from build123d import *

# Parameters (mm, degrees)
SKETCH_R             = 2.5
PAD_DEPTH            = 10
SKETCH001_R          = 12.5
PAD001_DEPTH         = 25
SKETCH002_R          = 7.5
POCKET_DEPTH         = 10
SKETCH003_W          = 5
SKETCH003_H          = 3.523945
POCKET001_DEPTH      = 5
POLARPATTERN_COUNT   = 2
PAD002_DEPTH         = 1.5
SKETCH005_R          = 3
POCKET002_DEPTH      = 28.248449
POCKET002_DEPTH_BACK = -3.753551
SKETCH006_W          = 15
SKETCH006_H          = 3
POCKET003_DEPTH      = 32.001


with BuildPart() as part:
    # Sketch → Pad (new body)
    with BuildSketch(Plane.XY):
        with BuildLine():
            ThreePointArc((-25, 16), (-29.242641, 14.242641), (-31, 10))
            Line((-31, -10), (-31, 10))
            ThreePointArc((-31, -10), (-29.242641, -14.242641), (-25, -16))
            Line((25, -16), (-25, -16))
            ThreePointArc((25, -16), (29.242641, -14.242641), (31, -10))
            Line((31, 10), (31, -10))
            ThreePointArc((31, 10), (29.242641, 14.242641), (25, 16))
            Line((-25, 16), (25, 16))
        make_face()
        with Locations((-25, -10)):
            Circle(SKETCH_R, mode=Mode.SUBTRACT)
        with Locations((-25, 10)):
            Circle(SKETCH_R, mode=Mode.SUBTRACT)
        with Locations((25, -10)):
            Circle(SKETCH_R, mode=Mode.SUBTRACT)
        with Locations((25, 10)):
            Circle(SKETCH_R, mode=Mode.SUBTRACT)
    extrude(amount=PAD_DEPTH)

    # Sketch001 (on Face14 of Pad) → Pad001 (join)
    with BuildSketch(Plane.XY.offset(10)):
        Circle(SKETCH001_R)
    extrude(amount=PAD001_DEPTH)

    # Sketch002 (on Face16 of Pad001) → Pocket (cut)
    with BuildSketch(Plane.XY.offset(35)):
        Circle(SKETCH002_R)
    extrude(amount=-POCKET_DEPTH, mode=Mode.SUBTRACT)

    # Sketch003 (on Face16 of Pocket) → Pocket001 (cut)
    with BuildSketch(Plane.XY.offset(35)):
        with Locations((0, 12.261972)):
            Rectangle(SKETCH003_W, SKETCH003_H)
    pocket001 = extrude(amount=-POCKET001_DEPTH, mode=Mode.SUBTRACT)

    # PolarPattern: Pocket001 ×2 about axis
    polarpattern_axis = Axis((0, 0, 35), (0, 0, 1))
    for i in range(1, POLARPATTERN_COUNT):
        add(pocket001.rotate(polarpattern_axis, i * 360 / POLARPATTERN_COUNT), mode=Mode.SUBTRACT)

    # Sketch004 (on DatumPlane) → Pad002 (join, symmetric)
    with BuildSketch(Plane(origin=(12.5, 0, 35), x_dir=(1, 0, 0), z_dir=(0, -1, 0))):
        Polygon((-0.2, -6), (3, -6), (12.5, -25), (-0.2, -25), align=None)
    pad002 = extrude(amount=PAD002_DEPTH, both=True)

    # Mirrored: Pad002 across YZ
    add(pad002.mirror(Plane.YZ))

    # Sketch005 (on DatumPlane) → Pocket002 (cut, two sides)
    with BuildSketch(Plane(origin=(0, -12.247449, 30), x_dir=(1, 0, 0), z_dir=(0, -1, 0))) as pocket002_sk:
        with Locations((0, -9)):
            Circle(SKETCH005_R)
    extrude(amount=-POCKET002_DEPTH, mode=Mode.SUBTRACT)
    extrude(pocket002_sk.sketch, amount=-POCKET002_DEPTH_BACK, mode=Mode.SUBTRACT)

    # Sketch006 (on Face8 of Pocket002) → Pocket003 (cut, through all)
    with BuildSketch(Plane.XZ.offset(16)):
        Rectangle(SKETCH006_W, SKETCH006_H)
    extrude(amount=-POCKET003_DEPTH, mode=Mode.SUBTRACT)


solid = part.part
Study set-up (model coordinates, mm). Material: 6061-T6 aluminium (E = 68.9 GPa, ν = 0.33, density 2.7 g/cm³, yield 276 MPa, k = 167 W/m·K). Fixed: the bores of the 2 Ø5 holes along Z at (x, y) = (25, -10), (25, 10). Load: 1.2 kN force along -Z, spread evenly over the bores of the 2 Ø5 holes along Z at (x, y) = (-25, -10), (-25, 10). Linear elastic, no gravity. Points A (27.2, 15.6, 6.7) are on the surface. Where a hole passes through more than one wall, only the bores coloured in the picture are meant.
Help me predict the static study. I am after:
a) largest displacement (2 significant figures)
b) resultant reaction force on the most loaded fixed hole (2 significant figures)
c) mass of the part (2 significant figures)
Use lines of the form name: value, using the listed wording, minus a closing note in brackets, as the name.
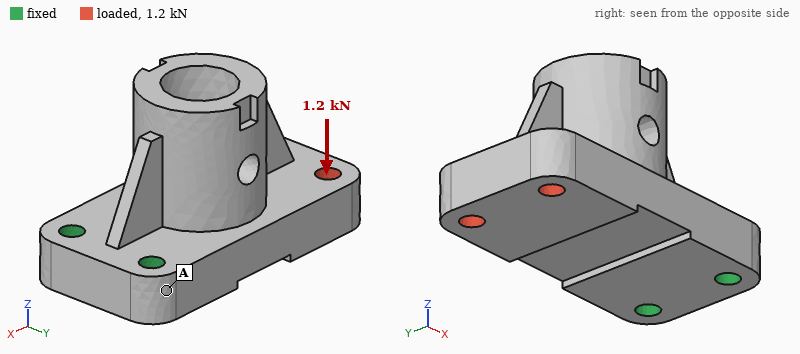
largest displacement: 0.22 mm
resultant reaction force on the most loaded fixed hole: 630 N
mass of the part: 77 g
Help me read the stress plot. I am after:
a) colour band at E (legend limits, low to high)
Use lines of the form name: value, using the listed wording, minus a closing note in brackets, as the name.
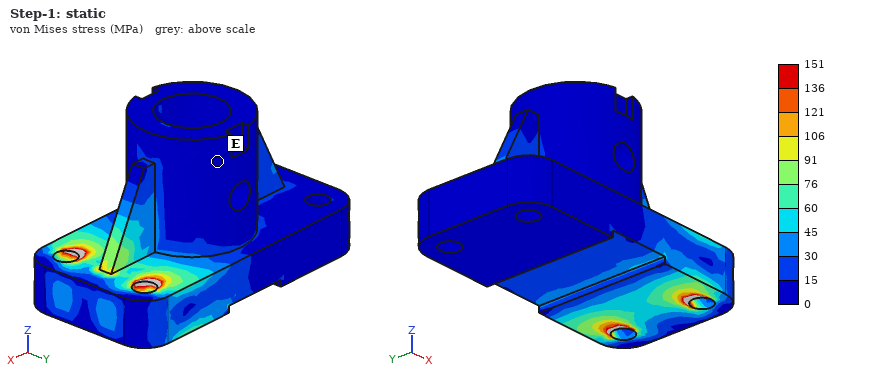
colour band at E: 0 to 15 MPa
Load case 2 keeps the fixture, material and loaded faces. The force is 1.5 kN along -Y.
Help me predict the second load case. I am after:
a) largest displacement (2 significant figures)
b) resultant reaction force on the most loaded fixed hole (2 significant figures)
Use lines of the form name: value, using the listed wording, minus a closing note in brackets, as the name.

largest displacement: 55 µm
resultant reaction force on the most loaded fixed hole: 3.4 kN
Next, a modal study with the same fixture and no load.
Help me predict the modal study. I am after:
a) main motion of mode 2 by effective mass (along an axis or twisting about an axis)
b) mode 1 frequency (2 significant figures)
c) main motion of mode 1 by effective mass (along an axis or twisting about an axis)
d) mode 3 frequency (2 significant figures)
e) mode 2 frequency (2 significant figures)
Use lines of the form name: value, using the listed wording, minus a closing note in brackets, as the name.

main motion of mode 2 by effective mass: along Y
mode 1 frequency: 2500 Hz
main motion of mode 1 by effective mass: along Z
mode 3 frequency: 6900 Hz
mode 2 frequency: 5600 Hz
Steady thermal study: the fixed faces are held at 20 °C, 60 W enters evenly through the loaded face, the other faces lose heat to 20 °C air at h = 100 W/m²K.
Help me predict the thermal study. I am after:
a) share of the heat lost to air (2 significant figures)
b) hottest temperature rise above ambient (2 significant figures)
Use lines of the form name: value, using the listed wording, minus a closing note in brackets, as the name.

share of the heat lost to air: 28 %
hottest temperature rise above ambient: 44 K
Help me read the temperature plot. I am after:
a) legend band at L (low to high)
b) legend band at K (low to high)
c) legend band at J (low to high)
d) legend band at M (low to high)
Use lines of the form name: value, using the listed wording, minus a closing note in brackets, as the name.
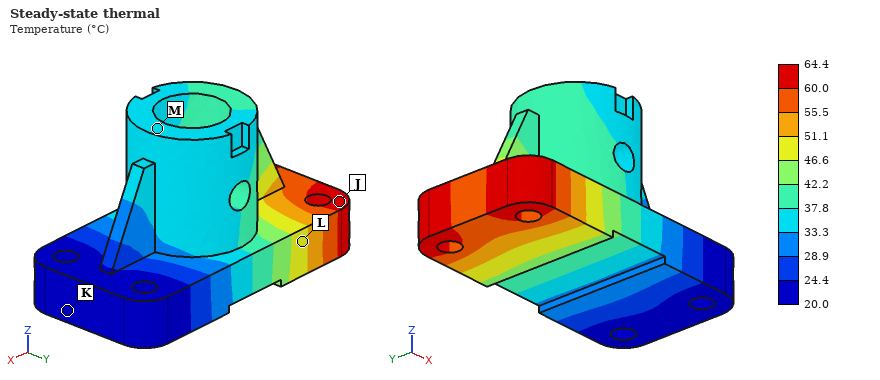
legend band at L: 46.6 to 51.1 °C
legend band at K: 20.0 to 24.4 °C
legend band at J: 60.0 to 64.4 °C
legend band at M: 33.3 to 37.8 °C
